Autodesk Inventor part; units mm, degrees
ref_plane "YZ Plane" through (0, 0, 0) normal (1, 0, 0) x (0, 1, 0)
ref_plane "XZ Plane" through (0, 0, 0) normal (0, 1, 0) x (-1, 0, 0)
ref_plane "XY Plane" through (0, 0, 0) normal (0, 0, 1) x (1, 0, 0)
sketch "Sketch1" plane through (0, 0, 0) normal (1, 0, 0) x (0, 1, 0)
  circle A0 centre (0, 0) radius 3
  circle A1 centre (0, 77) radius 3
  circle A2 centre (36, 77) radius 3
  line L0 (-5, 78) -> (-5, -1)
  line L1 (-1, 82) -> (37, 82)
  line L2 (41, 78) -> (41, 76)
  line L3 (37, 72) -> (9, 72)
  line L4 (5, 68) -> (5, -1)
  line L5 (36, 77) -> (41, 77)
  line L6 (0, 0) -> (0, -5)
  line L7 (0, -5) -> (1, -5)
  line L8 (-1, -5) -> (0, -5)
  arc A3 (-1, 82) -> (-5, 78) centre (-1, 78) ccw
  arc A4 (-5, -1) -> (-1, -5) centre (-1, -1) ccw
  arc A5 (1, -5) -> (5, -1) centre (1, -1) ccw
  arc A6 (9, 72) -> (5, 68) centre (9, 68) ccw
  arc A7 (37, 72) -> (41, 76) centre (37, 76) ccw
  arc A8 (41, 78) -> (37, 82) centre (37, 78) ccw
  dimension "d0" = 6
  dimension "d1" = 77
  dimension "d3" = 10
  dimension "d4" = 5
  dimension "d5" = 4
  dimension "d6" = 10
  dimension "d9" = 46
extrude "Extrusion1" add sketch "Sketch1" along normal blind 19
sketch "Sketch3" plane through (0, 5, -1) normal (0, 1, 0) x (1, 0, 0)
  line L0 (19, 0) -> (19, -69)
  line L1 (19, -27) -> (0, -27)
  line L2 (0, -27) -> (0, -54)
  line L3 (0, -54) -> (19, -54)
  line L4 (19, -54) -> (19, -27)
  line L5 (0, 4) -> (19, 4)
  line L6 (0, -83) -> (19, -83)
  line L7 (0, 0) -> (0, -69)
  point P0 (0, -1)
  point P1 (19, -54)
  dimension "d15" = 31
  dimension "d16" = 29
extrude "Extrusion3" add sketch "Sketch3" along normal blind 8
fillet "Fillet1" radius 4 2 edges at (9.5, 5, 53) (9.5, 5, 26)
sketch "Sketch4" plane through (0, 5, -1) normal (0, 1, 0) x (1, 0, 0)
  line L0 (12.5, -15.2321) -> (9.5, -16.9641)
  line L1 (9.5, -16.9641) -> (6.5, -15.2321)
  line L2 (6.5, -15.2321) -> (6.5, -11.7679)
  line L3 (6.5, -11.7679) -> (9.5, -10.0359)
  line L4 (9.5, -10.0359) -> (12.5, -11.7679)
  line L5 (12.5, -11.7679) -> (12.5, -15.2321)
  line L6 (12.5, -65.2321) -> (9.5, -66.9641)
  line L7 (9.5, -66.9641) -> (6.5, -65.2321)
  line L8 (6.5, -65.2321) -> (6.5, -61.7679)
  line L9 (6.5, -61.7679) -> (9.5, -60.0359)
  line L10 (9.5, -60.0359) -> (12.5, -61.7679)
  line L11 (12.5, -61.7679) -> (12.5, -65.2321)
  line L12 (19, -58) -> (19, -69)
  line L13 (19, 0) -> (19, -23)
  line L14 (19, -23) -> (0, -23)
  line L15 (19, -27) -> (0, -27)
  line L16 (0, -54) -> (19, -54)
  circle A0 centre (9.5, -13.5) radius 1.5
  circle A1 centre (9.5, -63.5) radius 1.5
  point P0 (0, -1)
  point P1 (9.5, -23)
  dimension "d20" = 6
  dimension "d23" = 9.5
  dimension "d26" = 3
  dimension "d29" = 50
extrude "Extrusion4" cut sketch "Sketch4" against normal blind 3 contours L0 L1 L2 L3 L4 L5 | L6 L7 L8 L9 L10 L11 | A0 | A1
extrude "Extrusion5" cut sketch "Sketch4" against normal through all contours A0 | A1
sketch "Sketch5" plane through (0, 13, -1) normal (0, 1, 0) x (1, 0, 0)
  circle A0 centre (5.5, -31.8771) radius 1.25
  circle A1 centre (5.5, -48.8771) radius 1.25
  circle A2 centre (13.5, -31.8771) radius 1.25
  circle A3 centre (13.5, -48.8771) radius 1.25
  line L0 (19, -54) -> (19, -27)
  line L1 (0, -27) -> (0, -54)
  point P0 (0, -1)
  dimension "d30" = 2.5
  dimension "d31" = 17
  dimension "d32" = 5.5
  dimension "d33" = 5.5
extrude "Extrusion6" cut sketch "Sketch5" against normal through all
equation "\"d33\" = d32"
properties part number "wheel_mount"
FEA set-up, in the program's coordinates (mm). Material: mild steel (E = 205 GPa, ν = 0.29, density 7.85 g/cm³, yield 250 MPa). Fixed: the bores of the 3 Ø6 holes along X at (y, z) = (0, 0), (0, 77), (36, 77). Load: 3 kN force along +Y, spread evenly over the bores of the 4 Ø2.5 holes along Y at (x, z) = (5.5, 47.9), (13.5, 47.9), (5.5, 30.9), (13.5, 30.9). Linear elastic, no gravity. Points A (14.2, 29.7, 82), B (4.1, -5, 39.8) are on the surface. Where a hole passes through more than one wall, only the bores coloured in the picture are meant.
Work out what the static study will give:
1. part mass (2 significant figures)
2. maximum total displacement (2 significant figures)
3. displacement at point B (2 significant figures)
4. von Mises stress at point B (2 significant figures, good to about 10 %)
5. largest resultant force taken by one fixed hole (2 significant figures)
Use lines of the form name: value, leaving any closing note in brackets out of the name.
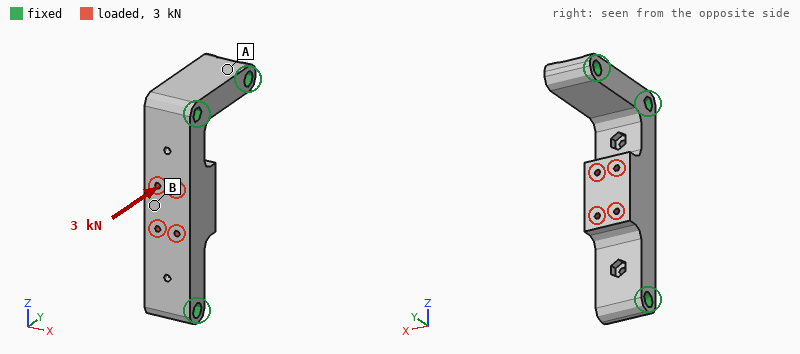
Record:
part mass: 200 g
maximum total displacement: 12 µm
displacement at point B: 12 µm
von Mises stress at point B: 18 MPa
largest resultant force taken by one fixed hole: 1.6 kN
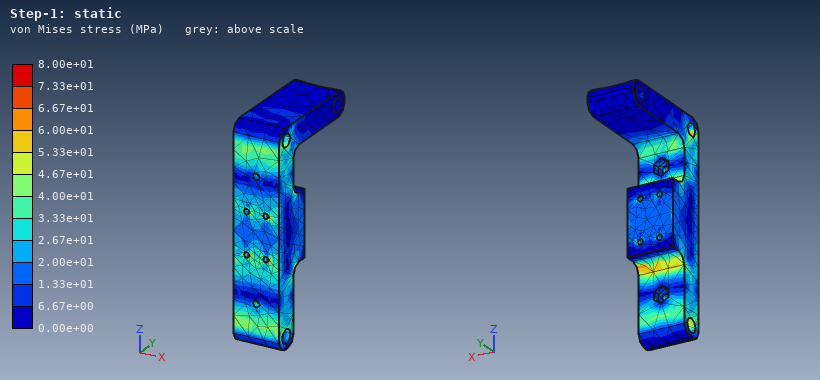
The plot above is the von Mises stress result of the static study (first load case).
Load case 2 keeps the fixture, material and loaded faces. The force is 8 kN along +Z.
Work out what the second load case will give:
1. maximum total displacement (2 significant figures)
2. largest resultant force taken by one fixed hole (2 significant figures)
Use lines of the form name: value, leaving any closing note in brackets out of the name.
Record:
maximum total displacement: 5.4 µm
largest resultant force taken by one fixed hole: 4.1 kN
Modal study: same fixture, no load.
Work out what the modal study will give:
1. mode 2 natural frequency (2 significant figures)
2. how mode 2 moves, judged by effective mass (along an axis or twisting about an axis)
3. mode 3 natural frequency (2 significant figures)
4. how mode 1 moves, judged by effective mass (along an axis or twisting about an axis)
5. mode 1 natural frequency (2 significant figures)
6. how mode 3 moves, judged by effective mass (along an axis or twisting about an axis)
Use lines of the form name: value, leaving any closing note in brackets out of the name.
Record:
mode 2 natural frequency: 9200 Hz
how mode 2 moves, judged by effective mass: along X
mode 3 natural frequency: 15 kHz
how mode 1 moves, judged by effective mass: along Y
mode 1 natural frequency: 8600 Hz
how mode 3 moves, judged by effective mass: along X
